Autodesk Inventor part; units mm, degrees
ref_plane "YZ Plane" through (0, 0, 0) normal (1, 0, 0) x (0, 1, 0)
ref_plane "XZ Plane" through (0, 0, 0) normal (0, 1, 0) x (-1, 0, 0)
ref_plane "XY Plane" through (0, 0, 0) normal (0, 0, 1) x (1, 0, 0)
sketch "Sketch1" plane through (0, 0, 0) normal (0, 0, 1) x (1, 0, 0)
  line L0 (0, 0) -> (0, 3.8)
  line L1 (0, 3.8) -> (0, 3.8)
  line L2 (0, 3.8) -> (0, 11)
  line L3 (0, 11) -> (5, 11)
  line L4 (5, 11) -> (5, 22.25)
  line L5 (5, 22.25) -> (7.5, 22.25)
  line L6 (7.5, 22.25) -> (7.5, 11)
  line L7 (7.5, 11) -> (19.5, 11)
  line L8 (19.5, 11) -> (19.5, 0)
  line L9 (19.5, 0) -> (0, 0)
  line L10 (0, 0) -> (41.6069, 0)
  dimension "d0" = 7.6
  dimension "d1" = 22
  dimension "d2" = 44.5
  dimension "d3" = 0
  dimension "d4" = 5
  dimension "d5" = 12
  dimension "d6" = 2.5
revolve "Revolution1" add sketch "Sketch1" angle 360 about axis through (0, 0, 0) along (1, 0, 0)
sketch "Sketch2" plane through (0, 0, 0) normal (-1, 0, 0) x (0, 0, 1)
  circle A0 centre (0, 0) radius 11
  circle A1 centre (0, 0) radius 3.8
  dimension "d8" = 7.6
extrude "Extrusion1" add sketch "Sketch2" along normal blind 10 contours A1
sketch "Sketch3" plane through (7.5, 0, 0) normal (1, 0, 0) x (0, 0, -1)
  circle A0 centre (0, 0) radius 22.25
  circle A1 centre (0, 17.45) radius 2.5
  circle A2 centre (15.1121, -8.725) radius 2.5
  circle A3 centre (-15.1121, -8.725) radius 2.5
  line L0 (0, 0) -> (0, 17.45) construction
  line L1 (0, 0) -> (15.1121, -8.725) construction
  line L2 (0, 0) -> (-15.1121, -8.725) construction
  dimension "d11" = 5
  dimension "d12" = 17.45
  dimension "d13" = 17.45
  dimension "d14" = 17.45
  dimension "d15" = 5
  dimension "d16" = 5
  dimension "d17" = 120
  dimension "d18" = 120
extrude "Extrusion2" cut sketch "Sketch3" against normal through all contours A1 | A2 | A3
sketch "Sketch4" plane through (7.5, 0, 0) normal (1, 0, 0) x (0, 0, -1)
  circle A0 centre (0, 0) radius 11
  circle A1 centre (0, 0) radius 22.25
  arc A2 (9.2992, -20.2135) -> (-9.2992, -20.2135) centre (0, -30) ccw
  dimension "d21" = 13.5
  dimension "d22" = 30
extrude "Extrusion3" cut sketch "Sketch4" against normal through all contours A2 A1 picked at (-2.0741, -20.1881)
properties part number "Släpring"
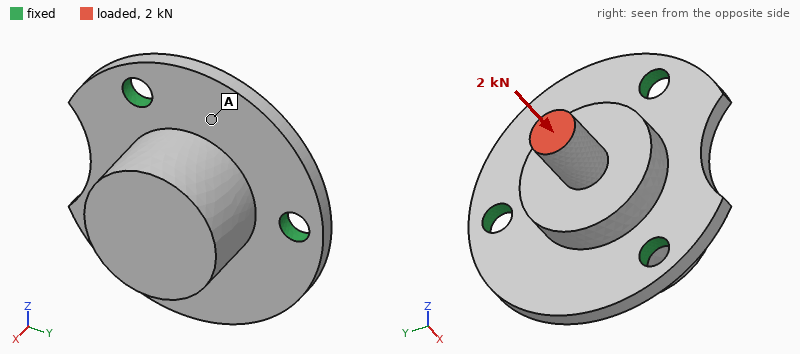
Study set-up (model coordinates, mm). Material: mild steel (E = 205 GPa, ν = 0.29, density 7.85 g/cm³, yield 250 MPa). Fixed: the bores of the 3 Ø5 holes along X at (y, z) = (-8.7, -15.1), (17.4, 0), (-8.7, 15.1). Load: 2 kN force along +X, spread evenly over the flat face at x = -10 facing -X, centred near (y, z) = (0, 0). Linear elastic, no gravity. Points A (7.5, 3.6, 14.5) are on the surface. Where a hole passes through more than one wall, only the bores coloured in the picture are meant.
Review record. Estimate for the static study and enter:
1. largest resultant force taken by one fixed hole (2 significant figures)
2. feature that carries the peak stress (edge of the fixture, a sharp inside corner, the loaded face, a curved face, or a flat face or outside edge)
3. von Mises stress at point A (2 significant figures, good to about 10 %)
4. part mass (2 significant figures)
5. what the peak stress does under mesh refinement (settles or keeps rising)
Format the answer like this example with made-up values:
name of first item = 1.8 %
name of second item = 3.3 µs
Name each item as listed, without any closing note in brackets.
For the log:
largest resultant force taken by one fixed hole = 670 N
feature that carries the peak stress = edge of the fixture
von Mises stress at point A = 17 MPa
part mass = 82 g
what the peak stress does under mesh refinement = keeps rising
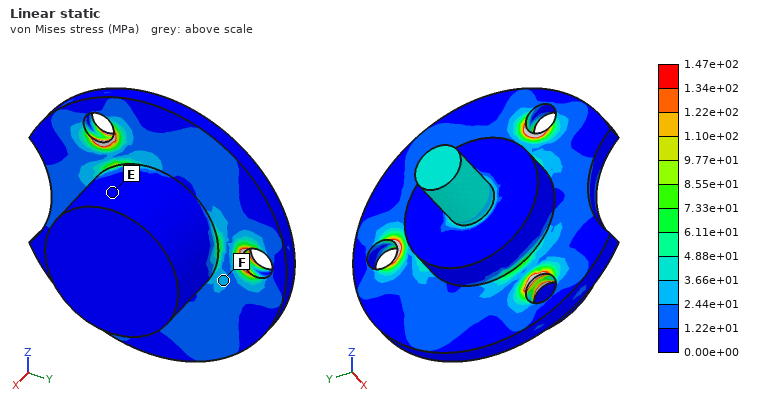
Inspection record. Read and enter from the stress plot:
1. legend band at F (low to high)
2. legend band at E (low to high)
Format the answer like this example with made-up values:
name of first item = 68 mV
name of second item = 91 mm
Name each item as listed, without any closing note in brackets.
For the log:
legend band at F = 2.44e+01 to 3.66e+01 MPa
legend band at E = 0.00e+00 to 1.22e+01 MPa
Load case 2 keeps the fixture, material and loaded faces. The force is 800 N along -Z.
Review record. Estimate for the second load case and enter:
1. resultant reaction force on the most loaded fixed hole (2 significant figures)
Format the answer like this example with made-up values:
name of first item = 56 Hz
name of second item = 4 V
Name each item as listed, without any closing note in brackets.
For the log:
resultant reaction force on the most loaded fixed hole = 590 N
